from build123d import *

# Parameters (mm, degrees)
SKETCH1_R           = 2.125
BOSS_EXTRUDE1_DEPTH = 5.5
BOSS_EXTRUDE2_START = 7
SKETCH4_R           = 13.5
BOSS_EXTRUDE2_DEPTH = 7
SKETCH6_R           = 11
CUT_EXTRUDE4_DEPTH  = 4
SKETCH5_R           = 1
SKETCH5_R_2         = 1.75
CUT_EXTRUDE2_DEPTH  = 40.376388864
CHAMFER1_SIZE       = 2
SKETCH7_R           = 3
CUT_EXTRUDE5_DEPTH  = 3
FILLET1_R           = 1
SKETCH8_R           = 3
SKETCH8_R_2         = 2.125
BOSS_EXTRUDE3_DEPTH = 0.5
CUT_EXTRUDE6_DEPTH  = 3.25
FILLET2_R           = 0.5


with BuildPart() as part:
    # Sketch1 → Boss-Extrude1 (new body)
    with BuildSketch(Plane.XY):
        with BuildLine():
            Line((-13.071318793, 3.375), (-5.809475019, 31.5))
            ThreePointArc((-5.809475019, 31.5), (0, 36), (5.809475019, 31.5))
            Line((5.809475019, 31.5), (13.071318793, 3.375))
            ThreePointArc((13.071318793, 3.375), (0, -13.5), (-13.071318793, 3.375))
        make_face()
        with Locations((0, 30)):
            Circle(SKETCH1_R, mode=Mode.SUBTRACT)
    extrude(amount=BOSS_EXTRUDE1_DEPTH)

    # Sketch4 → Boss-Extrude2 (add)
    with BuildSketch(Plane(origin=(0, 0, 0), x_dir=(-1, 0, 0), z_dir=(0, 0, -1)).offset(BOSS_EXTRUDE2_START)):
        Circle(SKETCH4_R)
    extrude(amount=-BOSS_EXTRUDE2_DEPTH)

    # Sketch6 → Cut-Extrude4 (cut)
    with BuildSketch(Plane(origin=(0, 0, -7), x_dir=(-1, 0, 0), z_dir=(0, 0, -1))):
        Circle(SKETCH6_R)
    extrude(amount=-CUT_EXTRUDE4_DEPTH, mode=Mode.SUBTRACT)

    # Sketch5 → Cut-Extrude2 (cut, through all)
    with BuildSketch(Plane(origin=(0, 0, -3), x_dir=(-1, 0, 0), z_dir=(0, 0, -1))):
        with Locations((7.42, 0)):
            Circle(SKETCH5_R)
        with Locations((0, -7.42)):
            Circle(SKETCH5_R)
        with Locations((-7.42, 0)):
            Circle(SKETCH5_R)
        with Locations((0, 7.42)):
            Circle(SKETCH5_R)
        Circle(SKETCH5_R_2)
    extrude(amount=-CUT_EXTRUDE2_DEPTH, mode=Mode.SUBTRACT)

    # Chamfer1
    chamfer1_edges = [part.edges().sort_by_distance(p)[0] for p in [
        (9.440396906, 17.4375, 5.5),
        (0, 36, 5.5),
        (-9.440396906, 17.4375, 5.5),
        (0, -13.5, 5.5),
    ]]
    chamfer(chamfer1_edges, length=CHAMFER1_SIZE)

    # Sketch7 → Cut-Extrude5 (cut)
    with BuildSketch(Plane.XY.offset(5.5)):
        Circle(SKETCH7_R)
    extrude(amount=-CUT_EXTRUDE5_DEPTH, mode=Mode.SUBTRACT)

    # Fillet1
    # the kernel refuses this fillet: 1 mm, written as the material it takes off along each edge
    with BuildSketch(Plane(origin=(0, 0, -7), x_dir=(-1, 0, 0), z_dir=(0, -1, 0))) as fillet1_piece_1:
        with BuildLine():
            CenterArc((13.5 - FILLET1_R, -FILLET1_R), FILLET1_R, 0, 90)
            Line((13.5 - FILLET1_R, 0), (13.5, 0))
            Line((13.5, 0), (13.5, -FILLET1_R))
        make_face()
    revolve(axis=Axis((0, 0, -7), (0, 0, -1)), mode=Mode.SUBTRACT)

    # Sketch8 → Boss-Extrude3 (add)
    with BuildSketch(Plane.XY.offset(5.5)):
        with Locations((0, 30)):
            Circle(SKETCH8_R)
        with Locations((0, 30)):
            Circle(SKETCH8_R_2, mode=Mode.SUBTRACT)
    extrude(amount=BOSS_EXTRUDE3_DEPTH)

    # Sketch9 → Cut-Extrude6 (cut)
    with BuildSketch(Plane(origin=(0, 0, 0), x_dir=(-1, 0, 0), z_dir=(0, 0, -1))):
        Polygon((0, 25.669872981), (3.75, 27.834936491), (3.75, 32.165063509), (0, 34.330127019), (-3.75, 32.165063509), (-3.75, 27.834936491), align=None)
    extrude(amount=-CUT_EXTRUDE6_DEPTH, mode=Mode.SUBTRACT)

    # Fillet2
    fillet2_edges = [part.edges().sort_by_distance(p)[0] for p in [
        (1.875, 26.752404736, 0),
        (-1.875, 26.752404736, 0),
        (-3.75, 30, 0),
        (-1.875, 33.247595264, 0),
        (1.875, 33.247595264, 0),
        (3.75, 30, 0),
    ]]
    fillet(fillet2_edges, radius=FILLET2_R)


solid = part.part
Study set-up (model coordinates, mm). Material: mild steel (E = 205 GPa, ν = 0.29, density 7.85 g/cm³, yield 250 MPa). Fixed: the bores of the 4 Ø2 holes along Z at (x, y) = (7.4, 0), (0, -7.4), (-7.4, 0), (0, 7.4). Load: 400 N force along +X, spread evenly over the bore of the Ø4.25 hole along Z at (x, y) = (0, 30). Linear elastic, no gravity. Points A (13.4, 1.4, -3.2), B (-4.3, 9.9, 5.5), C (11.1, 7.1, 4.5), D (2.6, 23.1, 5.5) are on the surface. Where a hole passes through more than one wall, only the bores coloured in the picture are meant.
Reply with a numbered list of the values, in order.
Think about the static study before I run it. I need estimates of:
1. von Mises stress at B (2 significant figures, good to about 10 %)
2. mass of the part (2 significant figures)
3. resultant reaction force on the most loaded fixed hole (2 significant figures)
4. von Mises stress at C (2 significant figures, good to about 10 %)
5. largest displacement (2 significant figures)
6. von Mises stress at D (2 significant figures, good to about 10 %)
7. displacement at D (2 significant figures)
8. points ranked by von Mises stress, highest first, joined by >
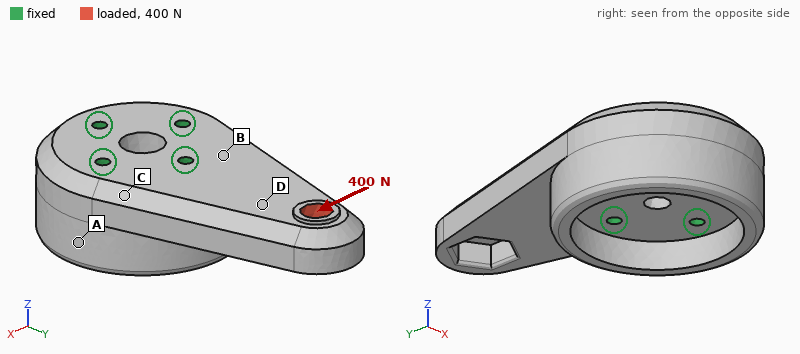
1. 8.2 MPa
2. 55 g
3. 470 N
4. 12 MPa
5. 6.2 µm
6. 17 MPa
7. 2.7 µm
8. D > C > B > A
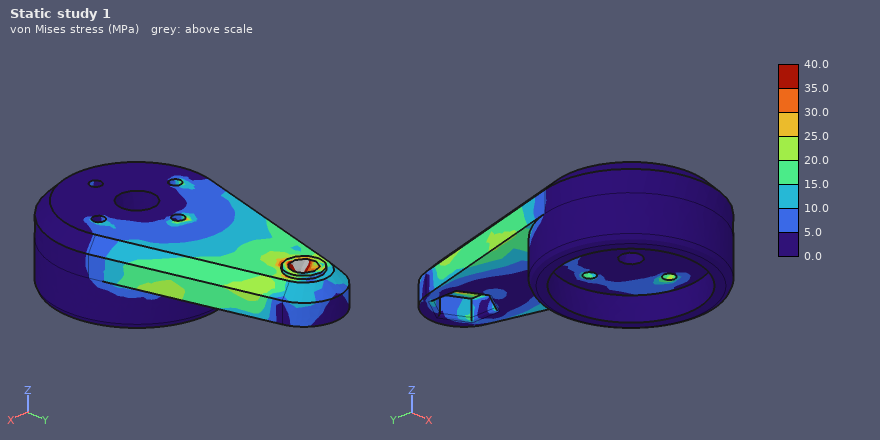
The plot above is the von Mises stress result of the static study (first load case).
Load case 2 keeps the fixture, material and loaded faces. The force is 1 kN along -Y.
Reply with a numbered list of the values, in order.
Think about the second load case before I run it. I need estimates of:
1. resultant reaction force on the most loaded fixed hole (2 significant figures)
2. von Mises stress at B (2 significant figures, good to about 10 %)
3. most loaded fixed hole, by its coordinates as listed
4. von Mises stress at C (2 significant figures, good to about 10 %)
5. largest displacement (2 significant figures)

1. 540 N
2. 19 MPa
3. (0, 7.4)
4. 8.5 MPa
5. 16 µm
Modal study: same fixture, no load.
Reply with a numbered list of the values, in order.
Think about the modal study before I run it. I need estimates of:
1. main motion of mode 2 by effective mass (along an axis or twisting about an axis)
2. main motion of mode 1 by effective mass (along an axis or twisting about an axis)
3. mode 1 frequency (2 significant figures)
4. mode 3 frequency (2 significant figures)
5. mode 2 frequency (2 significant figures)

1. along X
2. along Z
3. 9500 Hz
4. 26 kHz
5. 20 kHz
